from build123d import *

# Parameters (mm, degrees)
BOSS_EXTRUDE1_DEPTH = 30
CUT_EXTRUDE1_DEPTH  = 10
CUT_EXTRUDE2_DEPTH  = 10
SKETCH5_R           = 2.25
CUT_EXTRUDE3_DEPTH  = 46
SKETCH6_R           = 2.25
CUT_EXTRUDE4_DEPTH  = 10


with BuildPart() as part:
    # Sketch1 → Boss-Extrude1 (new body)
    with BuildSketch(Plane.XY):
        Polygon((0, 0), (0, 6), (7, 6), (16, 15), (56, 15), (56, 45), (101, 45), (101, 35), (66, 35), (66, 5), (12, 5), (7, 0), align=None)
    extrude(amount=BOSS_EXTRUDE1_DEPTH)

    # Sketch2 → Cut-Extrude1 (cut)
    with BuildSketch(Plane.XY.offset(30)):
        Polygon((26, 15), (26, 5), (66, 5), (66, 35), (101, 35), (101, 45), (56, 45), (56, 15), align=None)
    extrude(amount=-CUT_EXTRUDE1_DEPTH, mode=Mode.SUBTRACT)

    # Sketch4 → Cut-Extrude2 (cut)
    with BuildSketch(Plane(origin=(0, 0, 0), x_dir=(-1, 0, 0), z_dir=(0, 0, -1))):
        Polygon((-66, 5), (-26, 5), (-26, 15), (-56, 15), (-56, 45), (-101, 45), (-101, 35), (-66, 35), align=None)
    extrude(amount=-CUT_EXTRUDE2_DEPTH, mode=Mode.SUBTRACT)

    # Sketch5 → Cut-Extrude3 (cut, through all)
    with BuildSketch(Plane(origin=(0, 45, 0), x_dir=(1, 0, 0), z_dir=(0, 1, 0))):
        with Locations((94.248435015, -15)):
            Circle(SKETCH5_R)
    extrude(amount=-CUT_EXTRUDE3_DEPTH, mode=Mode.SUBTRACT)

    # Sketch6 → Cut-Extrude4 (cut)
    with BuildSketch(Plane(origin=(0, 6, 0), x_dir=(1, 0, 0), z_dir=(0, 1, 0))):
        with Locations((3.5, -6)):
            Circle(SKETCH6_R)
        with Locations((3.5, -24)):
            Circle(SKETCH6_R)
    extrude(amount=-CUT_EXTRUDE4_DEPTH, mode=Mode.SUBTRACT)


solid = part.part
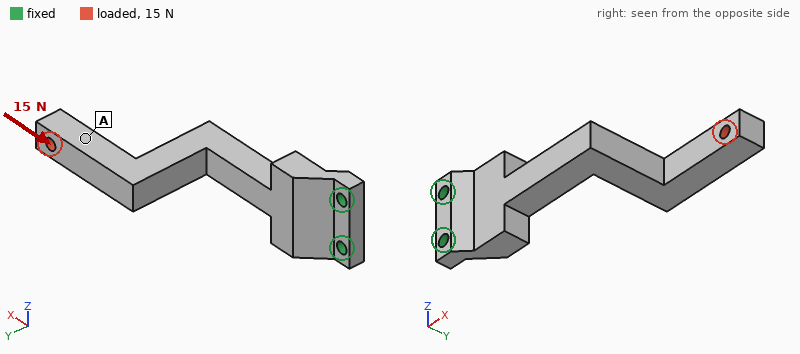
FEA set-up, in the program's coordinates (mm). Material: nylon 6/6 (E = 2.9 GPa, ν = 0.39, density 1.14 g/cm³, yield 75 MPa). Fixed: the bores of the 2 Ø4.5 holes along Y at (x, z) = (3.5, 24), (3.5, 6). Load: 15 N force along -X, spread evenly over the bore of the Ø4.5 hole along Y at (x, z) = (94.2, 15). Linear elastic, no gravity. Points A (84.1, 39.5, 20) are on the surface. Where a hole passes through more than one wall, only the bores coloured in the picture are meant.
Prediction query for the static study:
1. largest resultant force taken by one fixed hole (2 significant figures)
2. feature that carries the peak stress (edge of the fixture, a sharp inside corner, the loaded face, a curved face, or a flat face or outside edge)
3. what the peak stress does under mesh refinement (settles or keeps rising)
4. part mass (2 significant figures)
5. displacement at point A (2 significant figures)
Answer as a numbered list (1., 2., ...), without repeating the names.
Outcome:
1. 7.5 N
2. a sharp inside corner
3. keeps rising
4. 19 g
5. 1.1 mm
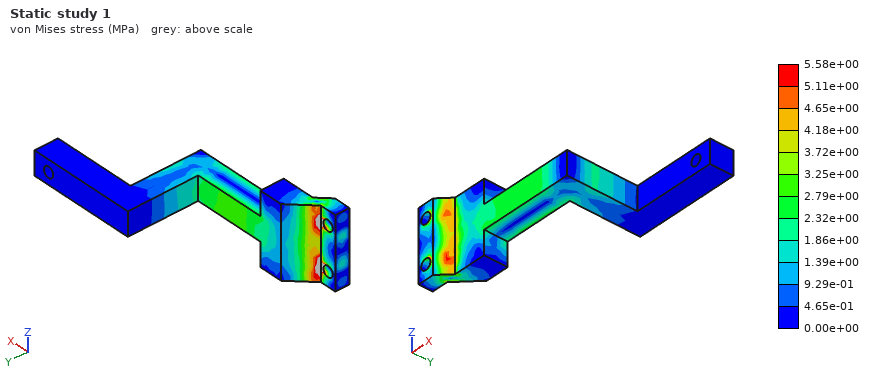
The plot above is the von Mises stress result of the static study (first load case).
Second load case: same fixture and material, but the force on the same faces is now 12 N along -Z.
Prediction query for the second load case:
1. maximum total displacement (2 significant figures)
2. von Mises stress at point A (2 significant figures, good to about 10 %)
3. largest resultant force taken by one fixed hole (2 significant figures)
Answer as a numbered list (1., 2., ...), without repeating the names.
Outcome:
1. 1.3 mm
2. 0.73 MPa
3. 57 N
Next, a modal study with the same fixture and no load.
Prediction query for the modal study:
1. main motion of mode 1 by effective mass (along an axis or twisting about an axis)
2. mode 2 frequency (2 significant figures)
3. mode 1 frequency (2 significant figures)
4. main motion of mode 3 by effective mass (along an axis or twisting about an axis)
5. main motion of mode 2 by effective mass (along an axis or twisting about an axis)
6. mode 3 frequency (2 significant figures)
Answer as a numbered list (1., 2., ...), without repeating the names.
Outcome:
1. along Y
2. 280 Hz
3. 170 Hz
4. along Y
5. along Z
6. 830 Hz
